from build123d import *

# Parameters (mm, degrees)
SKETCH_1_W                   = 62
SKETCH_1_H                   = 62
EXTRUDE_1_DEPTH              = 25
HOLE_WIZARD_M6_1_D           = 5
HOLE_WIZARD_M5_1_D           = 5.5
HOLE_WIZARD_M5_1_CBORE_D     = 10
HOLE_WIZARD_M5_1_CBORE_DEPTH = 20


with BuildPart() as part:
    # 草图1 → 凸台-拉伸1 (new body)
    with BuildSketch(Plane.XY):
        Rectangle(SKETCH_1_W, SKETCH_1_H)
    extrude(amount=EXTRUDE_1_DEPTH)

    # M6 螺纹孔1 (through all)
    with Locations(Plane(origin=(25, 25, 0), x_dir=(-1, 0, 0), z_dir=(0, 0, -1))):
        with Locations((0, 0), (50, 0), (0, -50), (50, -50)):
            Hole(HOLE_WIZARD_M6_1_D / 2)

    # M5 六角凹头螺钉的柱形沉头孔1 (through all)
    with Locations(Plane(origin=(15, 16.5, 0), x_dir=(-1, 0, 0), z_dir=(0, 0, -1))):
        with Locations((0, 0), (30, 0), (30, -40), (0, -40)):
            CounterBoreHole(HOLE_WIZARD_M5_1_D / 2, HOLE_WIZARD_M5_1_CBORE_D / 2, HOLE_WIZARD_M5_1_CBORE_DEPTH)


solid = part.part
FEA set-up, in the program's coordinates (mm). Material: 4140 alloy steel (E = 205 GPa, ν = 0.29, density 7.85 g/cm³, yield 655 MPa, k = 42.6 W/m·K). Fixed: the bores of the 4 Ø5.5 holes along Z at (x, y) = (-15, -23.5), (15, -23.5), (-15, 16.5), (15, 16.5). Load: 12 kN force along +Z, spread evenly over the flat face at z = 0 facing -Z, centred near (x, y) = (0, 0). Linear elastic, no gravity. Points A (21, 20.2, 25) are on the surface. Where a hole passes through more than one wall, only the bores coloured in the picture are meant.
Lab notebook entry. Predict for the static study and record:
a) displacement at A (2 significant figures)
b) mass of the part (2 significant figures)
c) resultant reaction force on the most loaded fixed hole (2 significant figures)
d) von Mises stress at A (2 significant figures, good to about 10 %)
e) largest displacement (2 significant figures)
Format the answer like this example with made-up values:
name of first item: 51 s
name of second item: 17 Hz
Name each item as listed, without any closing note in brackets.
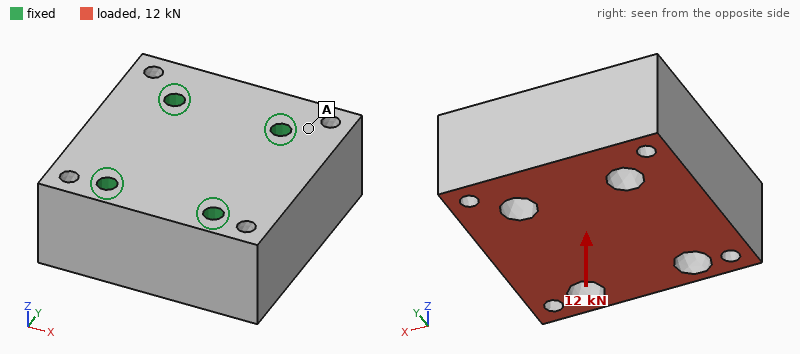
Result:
displacement at A: 1.7 µm
mass of the part: 690 g
resultant reaction force on the most loaded fixed hole: 3.6 kN
von Mises stress at A: 15 MPa
largest displacement: 2.8 µm
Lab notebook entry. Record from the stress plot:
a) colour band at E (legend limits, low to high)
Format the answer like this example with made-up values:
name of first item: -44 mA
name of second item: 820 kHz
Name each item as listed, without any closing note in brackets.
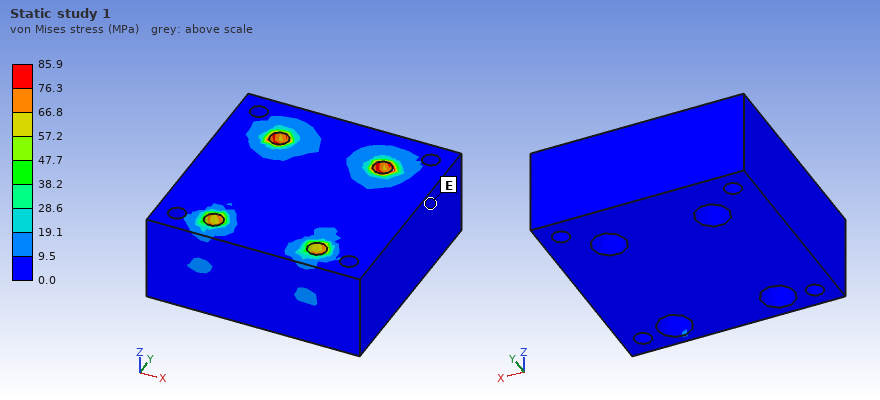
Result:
colour band at E: 0.0 to 9.5 MPa
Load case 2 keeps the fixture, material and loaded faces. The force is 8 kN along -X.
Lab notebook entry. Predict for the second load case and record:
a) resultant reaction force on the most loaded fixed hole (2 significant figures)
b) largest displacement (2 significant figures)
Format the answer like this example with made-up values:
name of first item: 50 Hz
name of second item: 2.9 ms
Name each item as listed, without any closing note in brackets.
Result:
resultant reaction force on the most loaded fixed hole: 3.7 kN
largest displacement: 6.9 µm
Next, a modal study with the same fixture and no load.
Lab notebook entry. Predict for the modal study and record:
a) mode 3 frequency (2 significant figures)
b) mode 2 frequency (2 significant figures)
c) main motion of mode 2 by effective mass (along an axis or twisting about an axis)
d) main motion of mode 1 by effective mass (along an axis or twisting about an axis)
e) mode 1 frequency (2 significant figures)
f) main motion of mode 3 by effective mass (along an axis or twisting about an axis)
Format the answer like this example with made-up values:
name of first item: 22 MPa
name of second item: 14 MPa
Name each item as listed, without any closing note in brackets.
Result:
mode 3 frequency: 15 kHz
mode 2 frequency: 13 kHz
main motion of mode 2 by effective mass: along Y
main motion of mode 1 by effective mass: along X
mode 1 frequency: 9900 Hz
main motion of mode 3 by effective mass: along Z
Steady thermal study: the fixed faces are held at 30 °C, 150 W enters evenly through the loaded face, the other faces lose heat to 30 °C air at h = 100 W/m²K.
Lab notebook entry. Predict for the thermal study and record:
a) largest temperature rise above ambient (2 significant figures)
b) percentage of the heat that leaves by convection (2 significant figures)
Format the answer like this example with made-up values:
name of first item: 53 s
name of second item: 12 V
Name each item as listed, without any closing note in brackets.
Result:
largest temperature rise above ambient: 47 K
percentage of the heat that leaves by convection: 27 %
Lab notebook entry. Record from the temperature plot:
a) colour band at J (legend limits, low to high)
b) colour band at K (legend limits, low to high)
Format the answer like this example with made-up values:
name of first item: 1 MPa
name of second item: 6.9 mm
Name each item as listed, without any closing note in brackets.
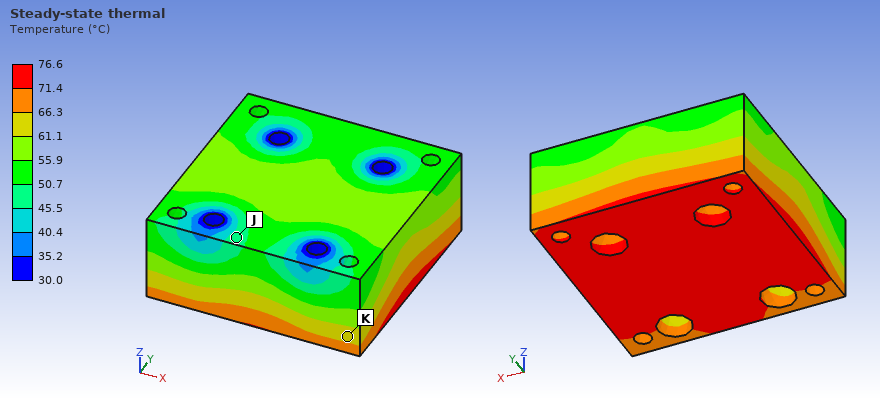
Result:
colour band at J: 45.5 to 50.7 °C
colour band at K: 61.1 to 66.3 °C
